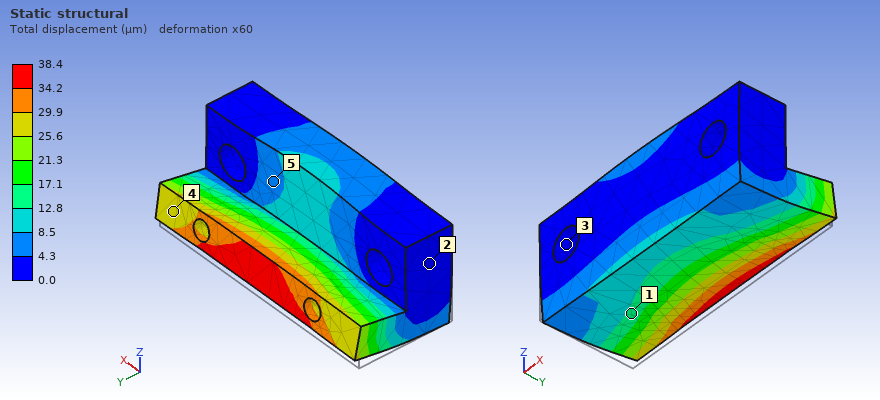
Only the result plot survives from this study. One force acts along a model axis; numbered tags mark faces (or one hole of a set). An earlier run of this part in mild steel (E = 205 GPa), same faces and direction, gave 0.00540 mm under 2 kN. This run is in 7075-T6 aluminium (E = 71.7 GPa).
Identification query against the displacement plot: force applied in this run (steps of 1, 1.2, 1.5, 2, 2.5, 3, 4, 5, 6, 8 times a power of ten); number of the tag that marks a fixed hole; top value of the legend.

5 kN
3
38.4 µm
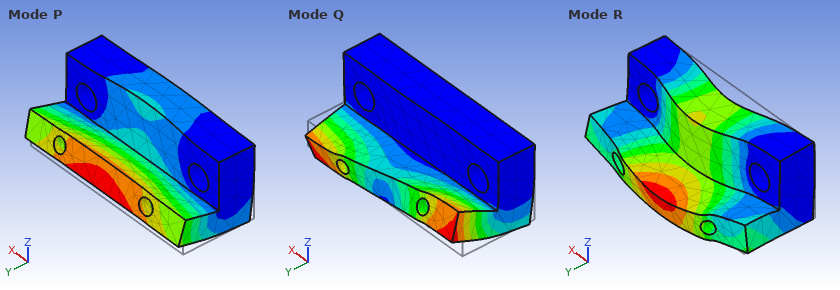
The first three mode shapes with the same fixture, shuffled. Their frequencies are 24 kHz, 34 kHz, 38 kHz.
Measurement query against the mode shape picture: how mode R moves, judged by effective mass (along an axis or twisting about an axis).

along Y
